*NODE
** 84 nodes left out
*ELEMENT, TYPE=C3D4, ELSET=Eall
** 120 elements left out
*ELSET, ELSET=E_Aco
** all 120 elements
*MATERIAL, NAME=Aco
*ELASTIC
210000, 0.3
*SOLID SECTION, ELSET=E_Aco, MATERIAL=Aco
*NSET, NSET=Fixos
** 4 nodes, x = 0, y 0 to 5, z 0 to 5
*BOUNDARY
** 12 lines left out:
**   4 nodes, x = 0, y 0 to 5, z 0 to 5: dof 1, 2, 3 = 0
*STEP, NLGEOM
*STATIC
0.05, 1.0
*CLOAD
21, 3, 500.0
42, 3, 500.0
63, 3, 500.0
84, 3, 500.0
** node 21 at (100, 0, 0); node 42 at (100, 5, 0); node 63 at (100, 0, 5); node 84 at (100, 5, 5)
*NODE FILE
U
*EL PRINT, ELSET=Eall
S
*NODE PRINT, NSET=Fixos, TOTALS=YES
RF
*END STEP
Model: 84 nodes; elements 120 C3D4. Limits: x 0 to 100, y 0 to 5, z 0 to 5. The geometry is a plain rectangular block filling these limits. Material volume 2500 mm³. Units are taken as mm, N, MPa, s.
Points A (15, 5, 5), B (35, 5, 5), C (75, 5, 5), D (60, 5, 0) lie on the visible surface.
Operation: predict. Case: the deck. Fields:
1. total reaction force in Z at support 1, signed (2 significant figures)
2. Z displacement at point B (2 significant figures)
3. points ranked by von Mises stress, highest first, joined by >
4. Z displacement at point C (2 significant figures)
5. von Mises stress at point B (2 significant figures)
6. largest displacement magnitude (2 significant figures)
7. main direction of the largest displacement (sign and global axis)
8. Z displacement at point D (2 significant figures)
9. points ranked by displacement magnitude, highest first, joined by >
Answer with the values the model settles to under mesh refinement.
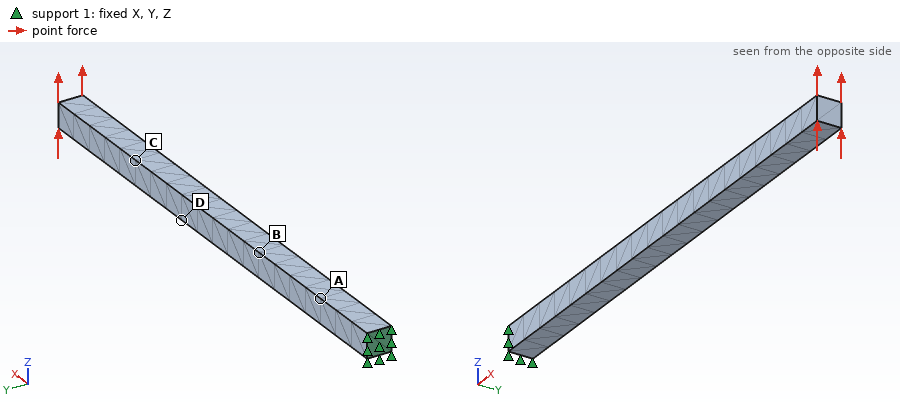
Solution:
-2000 N
7.9 mm
A > B > D > C
30 mm
4800 MPa
49 mm
+Z
21 mm
C > D > B > A
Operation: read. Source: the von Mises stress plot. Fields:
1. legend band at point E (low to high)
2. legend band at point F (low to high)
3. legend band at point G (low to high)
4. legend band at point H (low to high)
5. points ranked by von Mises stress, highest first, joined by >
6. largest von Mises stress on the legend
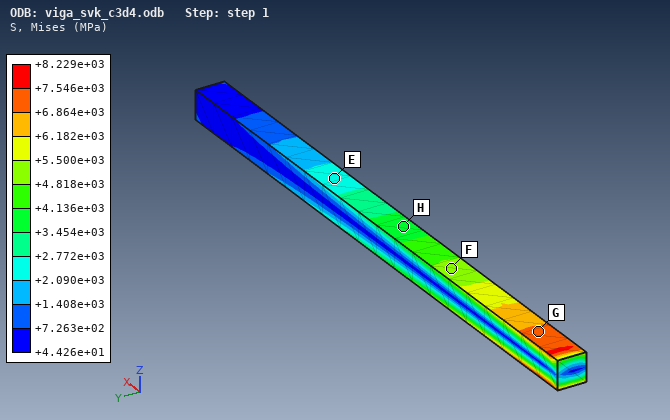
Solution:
+2.090e+03 to +2.772e+03 MPa
+4.818e+03 to +5.500e+03 MPa
+6.864e+03 to +7.546e+03 MPa
+3.454e+03 to +4.136e+03 MPa
G > F > H > E
+8.229e+03 MPa
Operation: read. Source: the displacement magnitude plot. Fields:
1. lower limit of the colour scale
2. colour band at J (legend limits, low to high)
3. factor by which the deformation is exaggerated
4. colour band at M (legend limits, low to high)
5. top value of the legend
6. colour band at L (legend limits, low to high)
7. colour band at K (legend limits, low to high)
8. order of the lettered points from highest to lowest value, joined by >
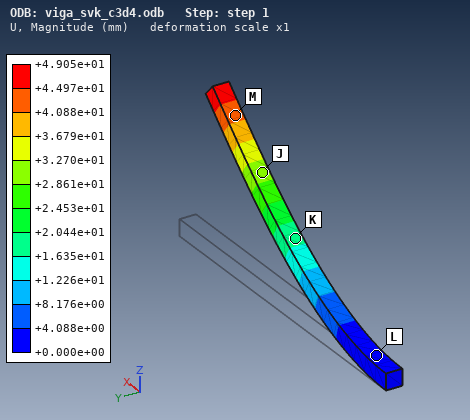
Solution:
+0.000e+00 mm
+2.861e+01 to +3.270e+01 mm
1
+4.088e+01 to +4.497e+01 mm
+4.905e+01 mm
+0.000e+00 to +4.088e+00 mm
+1.635e+01 to +2.044e+01 mm
M > J > K > L
